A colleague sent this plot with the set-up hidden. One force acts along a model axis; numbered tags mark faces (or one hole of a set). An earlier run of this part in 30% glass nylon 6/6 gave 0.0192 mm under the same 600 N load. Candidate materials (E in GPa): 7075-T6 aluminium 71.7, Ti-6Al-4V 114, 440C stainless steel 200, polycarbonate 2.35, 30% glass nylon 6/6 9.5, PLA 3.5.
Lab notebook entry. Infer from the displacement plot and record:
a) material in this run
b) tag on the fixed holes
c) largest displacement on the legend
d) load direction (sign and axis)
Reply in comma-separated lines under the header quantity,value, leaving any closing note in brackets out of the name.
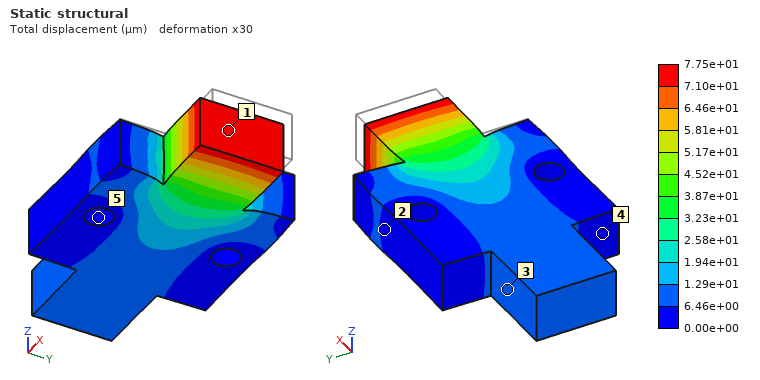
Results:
quantity,value
material in this run,polycarbonate
tag on the fixed holes,5
largest displacement on the legend,7.75e+01 µm
load direction,-X
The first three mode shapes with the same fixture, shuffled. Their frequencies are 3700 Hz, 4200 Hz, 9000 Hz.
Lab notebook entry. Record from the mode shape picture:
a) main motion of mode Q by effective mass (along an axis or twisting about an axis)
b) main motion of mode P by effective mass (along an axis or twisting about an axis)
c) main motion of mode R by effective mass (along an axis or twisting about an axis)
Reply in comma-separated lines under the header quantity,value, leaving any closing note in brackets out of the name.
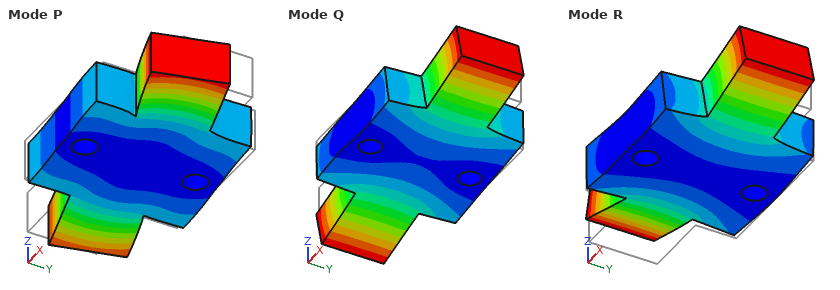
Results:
quantity,value
main motion of mode Q by effective mass,twisting about Y
main motion of mode P by effective mass,twisting about Z
main motion of mode R by effective mass,along Z
